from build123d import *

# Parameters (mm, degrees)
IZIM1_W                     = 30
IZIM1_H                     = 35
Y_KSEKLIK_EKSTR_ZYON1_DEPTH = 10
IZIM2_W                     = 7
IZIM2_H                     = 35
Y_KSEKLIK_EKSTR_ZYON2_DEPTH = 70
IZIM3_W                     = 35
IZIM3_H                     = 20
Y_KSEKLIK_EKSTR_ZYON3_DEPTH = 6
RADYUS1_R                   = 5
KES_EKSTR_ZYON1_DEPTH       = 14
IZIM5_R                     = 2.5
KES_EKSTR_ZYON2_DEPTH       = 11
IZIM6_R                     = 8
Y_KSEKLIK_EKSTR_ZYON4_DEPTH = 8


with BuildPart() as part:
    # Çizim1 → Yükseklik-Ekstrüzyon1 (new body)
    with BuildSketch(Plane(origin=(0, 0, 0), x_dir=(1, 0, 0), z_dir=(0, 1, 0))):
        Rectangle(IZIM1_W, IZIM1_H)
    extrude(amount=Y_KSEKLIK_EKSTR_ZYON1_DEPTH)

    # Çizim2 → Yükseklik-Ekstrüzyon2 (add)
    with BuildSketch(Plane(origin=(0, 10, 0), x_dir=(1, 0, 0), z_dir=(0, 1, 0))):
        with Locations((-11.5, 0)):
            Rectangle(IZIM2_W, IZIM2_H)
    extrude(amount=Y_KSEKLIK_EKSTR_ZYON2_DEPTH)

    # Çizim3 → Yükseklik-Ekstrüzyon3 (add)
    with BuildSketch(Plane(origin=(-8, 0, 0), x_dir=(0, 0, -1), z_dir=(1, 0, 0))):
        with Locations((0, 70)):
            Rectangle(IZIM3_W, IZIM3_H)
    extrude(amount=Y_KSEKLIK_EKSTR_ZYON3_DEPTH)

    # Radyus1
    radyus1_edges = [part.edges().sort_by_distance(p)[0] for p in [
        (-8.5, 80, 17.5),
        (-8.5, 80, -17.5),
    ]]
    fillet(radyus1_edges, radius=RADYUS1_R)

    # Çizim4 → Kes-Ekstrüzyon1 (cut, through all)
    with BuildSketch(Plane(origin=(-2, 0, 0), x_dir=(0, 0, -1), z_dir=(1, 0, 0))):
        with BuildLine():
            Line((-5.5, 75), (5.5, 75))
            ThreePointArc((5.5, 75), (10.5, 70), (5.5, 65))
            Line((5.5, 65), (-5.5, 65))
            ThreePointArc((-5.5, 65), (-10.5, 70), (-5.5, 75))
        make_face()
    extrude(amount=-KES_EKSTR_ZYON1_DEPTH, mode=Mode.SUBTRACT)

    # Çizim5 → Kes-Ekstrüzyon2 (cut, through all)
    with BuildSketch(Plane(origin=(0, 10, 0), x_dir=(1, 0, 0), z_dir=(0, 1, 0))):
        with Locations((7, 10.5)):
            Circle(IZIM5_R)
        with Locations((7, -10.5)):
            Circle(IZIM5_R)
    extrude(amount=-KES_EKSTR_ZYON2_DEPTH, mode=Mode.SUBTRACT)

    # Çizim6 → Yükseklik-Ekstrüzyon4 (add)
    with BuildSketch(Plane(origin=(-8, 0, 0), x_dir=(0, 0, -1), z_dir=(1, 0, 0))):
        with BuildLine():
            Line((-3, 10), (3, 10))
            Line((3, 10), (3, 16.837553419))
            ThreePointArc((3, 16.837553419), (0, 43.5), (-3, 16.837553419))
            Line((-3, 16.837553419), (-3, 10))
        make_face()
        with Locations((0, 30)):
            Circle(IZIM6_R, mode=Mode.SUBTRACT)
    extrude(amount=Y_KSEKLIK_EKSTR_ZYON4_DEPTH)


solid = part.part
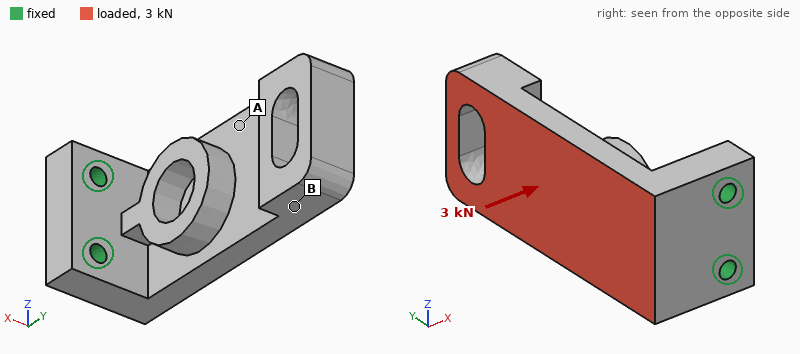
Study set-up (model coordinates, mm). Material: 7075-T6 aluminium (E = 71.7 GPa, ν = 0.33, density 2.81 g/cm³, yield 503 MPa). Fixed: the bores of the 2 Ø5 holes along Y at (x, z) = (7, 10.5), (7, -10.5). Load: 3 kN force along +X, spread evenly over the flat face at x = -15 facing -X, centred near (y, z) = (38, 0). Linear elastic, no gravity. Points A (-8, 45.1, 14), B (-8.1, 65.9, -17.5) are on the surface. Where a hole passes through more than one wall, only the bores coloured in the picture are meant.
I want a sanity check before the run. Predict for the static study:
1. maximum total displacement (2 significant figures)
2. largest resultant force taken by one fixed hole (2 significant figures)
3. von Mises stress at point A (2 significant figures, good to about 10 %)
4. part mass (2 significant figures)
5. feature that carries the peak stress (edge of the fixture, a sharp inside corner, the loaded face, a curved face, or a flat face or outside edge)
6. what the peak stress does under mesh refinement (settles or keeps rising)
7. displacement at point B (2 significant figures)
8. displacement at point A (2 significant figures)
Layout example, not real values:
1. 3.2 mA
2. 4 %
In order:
1. 1.1 mm
2. 1.7 kN
3. 54 MPa
4. 90 g
5. edge of the fixture
6. keeps rising
7. 0.83 mm
8. 0.46 mm
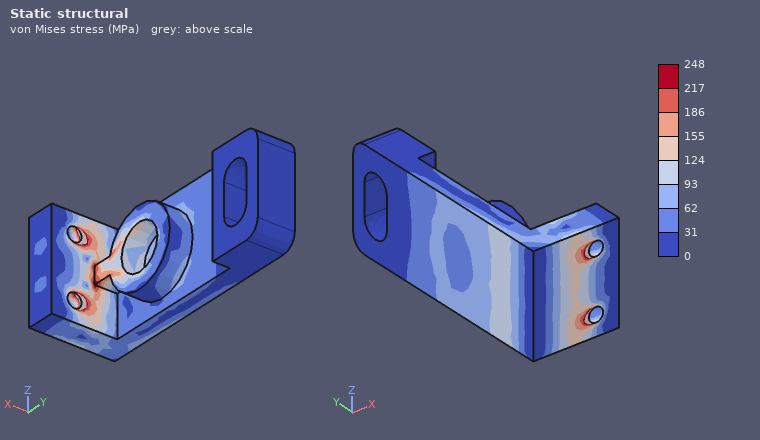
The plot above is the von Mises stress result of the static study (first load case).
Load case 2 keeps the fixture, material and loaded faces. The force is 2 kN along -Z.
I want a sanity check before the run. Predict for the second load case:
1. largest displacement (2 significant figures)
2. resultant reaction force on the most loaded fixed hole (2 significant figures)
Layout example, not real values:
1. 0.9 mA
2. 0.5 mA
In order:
1. 0.22 mm
2. 3.2 kN
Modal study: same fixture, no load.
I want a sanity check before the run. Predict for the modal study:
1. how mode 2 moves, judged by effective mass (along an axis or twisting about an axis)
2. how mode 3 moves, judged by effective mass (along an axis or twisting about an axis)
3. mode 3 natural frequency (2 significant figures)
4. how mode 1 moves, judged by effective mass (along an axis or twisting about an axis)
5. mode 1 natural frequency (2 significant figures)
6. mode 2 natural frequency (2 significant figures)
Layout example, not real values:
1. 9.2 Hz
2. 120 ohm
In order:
1. along Z
2. twisting about Y
3. 4600 Hz
4. along X
5. 1200 Hz
6. 2100 Hz
